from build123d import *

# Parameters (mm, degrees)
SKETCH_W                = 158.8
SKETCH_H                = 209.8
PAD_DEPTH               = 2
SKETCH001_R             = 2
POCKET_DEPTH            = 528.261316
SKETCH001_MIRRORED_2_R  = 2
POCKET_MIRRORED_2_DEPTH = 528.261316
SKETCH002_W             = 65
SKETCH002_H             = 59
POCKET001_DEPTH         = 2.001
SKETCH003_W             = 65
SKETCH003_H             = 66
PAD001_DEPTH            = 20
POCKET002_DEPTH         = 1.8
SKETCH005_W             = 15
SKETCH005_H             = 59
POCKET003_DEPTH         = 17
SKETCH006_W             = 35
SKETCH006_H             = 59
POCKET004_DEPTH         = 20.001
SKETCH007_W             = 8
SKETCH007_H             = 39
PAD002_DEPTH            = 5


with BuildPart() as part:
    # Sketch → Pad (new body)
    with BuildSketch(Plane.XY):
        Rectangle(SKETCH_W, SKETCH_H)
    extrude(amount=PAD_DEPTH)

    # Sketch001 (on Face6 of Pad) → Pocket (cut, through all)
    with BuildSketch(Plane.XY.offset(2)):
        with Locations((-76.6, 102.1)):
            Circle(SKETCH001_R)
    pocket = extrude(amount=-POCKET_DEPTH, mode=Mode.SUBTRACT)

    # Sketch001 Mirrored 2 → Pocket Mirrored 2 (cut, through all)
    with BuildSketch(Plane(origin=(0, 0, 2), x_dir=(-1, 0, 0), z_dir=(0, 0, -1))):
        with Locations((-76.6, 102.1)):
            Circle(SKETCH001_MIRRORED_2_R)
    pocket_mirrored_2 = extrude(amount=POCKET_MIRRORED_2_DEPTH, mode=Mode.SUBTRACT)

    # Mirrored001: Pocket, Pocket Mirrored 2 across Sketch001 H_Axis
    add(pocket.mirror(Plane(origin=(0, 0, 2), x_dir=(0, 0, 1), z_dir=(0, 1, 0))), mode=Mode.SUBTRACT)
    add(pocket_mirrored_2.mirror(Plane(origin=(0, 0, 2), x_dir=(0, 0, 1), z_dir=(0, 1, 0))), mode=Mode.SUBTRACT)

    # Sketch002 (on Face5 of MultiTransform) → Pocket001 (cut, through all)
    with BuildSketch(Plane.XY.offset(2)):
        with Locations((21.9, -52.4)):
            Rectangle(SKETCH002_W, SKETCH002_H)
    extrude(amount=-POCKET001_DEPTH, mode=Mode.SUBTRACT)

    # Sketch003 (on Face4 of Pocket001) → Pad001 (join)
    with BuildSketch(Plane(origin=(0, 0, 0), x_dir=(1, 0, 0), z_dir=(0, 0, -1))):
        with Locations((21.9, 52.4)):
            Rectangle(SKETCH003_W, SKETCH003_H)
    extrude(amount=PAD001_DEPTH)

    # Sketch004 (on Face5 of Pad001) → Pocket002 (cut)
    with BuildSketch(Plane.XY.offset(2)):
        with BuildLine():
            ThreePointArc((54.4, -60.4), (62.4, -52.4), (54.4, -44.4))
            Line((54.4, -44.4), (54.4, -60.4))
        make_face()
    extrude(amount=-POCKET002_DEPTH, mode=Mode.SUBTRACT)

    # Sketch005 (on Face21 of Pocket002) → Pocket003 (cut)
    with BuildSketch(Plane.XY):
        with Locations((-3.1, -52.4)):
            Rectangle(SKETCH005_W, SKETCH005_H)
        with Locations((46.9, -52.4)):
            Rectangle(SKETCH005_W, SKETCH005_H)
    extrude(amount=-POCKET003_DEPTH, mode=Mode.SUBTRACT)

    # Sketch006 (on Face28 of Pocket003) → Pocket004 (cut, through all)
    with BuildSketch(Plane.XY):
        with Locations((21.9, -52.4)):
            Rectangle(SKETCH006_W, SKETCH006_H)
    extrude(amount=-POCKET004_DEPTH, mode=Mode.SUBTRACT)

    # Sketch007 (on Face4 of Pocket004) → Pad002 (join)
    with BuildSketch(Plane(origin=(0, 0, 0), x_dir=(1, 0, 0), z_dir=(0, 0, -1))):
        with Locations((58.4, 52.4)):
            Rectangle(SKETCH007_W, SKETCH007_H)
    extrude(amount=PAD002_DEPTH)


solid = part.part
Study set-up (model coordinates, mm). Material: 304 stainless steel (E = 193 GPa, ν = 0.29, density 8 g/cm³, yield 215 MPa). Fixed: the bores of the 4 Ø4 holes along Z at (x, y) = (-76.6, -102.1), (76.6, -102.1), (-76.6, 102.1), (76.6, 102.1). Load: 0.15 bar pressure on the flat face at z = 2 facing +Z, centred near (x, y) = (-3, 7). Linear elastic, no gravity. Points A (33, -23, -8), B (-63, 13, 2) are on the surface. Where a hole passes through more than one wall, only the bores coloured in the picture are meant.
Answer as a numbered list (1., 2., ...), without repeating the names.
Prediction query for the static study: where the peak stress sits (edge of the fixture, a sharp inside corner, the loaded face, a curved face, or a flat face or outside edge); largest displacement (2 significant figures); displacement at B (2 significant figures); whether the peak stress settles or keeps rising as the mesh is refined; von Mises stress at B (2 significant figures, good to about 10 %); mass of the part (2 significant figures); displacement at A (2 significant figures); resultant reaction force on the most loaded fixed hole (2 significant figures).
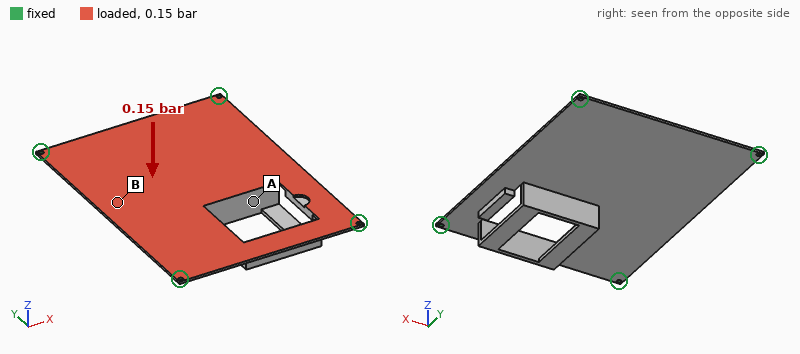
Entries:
1. edge of the fixture
2. 1.1 mm
3. 0.99 mm
4. keeps rising
5. 57 MPa
6. 600 g
7. 0.85 mm
8. 130 N
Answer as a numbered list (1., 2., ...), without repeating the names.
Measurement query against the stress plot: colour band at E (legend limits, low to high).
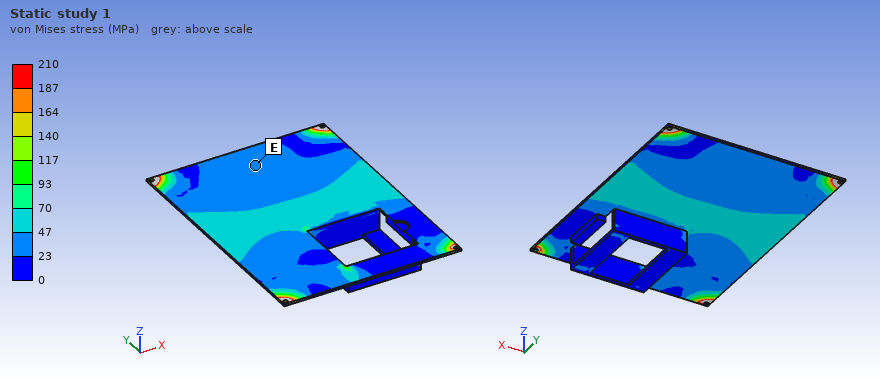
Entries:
1. 23 to 47 MPa
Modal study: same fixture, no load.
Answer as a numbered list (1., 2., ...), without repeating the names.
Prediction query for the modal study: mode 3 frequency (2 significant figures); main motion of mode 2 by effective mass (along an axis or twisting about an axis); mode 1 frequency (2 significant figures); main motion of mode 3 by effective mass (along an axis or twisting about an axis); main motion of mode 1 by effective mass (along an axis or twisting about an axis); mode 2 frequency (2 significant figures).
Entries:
1. 400 Hz
2. twisting about Y
3. 150 Hz
4. twisting about X
5. along Z
6. 310 Hz
